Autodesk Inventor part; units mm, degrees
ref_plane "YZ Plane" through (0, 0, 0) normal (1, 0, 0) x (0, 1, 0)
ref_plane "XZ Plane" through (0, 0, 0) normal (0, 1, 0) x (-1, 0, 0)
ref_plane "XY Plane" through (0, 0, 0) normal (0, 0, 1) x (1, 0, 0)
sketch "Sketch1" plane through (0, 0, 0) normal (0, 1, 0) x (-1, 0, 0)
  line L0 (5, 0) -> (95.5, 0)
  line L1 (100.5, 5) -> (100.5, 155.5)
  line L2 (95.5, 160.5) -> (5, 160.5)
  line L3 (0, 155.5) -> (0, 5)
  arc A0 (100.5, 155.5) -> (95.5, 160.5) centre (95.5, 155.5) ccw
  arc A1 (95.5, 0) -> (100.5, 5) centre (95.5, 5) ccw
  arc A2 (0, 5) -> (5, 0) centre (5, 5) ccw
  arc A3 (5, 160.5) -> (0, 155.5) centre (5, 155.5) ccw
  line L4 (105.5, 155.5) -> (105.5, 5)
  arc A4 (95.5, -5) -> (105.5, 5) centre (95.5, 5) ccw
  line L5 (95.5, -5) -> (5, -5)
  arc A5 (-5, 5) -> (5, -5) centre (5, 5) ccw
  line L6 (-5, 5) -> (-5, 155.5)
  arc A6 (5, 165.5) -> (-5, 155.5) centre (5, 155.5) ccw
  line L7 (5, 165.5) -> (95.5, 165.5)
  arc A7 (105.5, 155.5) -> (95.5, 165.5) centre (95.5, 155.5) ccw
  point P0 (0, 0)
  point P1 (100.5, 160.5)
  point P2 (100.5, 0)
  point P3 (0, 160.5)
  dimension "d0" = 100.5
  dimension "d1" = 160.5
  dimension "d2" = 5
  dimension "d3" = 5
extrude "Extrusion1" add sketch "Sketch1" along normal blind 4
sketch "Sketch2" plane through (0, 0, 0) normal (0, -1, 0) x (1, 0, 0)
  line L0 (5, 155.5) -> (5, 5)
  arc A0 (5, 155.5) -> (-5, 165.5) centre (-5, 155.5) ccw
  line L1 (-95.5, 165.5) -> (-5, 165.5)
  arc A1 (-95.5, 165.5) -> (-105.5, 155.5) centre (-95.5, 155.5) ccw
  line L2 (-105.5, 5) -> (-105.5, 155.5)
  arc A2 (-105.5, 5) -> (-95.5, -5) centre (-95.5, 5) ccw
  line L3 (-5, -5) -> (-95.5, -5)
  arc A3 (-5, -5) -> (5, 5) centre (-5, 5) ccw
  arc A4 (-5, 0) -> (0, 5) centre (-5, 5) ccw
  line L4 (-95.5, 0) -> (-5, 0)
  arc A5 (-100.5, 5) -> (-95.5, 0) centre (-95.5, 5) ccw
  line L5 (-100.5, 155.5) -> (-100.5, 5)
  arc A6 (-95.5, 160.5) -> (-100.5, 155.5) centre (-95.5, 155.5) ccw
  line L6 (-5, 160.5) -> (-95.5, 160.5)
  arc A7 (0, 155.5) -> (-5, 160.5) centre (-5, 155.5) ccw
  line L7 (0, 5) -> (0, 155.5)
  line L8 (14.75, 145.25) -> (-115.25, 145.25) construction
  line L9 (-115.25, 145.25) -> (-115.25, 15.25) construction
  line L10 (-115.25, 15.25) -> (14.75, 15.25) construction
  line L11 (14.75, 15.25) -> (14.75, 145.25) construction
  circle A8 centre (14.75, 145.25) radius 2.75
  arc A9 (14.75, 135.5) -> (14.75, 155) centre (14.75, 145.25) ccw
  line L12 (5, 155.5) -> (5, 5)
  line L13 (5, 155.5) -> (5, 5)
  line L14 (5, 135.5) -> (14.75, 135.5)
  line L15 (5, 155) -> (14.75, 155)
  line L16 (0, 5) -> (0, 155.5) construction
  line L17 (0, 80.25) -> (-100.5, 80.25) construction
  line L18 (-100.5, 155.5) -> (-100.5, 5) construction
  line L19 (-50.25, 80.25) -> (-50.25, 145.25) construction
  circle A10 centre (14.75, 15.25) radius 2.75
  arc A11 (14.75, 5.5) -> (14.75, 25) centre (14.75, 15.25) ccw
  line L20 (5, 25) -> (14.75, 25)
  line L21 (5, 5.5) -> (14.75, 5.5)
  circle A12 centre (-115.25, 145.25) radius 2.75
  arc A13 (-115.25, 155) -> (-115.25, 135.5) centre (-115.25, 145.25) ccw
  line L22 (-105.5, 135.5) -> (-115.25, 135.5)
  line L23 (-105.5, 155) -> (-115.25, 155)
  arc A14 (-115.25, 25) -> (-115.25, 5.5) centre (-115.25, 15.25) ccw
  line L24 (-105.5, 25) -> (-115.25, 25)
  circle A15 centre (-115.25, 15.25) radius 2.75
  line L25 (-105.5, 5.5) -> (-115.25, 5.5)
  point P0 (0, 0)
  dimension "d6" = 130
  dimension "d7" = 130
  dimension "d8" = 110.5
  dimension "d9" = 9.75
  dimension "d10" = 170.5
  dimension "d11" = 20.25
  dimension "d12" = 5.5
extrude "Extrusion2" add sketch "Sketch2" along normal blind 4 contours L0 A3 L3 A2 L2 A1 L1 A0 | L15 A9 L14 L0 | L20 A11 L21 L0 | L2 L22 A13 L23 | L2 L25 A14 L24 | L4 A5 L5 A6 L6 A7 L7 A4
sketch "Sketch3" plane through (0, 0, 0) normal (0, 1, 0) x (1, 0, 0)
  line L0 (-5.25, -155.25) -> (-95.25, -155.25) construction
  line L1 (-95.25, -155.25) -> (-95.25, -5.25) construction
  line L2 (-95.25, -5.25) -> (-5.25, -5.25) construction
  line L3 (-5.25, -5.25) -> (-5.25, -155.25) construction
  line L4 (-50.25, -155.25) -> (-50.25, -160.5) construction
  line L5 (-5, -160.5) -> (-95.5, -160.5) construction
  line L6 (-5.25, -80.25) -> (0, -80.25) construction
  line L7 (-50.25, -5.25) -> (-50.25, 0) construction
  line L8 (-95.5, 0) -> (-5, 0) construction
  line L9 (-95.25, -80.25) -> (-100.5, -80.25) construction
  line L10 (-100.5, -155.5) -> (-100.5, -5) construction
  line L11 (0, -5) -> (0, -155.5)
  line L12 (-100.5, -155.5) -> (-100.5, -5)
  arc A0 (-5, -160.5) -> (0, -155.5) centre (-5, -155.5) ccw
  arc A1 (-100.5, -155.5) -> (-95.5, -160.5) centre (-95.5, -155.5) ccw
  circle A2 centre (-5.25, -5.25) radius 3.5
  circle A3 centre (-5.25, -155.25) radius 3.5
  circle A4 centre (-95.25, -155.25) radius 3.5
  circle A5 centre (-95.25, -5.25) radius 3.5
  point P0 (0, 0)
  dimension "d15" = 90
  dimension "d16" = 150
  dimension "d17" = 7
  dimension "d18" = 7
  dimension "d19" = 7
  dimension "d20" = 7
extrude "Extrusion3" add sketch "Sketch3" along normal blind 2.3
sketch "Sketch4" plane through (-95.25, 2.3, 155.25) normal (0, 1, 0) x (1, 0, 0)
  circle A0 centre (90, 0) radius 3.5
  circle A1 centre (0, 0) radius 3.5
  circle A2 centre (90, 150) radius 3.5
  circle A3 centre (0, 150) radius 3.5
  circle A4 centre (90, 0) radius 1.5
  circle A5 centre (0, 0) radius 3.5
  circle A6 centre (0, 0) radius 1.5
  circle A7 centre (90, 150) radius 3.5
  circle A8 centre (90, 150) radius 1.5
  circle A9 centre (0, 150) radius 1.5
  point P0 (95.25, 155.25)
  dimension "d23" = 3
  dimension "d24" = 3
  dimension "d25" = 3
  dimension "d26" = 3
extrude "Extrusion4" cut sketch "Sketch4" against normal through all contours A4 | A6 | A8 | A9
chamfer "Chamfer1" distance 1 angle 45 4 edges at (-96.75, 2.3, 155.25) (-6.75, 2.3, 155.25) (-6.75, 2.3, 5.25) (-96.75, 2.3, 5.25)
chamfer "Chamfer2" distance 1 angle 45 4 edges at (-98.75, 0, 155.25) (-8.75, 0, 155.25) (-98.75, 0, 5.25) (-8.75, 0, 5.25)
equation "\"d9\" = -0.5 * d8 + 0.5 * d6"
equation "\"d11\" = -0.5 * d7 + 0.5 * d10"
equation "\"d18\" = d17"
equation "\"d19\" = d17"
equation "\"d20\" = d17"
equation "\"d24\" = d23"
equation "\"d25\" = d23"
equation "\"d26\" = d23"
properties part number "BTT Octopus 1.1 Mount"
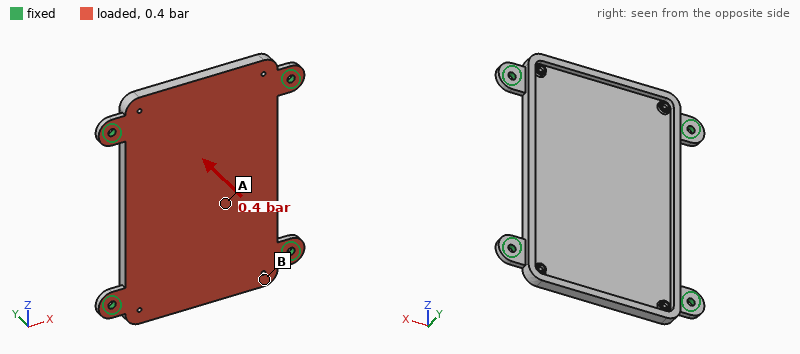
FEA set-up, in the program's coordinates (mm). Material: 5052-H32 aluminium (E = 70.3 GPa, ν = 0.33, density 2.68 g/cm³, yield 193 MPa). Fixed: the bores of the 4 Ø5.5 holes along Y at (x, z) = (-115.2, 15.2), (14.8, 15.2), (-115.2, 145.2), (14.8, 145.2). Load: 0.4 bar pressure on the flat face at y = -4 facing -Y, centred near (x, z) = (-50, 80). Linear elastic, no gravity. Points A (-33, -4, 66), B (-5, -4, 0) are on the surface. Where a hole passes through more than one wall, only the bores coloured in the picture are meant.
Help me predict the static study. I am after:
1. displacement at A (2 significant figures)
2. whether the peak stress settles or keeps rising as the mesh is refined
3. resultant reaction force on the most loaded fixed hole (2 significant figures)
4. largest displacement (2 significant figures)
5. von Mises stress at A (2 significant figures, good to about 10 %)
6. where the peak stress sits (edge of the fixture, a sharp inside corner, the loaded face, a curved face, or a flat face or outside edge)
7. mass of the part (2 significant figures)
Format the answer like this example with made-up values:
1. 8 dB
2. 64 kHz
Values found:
1. 0.17 mm
2. keeps rising
3. 220 N
4. 0.18 mm
5. 13 MPa
6. edge of the fixture
7. 240 g
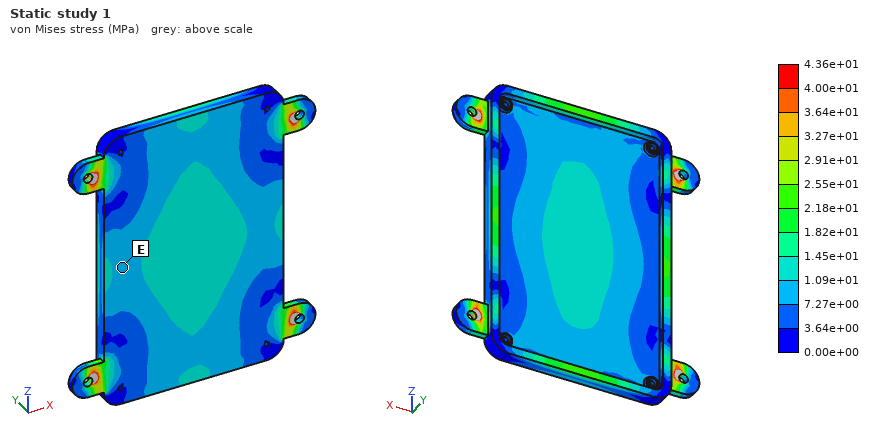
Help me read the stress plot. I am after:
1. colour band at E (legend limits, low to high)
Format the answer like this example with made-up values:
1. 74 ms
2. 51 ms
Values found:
1. 7.27e+00 to 1.09e+01 MPa
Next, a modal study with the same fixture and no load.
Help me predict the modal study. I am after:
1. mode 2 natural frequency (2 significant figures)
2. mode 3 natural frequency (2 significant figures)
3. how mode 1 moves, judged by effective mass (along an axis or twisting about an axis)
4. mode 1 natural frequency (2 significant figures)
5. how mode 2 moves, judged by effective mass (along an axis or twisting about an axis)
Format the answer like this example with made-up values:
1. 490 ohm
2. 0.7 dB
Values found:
1. 1400 Hz
2. 1500 Hz
3. along Y
4. 850 Hz
5. twisting about X
